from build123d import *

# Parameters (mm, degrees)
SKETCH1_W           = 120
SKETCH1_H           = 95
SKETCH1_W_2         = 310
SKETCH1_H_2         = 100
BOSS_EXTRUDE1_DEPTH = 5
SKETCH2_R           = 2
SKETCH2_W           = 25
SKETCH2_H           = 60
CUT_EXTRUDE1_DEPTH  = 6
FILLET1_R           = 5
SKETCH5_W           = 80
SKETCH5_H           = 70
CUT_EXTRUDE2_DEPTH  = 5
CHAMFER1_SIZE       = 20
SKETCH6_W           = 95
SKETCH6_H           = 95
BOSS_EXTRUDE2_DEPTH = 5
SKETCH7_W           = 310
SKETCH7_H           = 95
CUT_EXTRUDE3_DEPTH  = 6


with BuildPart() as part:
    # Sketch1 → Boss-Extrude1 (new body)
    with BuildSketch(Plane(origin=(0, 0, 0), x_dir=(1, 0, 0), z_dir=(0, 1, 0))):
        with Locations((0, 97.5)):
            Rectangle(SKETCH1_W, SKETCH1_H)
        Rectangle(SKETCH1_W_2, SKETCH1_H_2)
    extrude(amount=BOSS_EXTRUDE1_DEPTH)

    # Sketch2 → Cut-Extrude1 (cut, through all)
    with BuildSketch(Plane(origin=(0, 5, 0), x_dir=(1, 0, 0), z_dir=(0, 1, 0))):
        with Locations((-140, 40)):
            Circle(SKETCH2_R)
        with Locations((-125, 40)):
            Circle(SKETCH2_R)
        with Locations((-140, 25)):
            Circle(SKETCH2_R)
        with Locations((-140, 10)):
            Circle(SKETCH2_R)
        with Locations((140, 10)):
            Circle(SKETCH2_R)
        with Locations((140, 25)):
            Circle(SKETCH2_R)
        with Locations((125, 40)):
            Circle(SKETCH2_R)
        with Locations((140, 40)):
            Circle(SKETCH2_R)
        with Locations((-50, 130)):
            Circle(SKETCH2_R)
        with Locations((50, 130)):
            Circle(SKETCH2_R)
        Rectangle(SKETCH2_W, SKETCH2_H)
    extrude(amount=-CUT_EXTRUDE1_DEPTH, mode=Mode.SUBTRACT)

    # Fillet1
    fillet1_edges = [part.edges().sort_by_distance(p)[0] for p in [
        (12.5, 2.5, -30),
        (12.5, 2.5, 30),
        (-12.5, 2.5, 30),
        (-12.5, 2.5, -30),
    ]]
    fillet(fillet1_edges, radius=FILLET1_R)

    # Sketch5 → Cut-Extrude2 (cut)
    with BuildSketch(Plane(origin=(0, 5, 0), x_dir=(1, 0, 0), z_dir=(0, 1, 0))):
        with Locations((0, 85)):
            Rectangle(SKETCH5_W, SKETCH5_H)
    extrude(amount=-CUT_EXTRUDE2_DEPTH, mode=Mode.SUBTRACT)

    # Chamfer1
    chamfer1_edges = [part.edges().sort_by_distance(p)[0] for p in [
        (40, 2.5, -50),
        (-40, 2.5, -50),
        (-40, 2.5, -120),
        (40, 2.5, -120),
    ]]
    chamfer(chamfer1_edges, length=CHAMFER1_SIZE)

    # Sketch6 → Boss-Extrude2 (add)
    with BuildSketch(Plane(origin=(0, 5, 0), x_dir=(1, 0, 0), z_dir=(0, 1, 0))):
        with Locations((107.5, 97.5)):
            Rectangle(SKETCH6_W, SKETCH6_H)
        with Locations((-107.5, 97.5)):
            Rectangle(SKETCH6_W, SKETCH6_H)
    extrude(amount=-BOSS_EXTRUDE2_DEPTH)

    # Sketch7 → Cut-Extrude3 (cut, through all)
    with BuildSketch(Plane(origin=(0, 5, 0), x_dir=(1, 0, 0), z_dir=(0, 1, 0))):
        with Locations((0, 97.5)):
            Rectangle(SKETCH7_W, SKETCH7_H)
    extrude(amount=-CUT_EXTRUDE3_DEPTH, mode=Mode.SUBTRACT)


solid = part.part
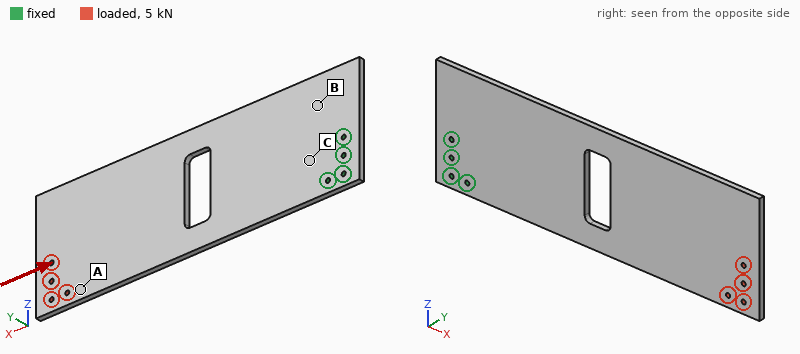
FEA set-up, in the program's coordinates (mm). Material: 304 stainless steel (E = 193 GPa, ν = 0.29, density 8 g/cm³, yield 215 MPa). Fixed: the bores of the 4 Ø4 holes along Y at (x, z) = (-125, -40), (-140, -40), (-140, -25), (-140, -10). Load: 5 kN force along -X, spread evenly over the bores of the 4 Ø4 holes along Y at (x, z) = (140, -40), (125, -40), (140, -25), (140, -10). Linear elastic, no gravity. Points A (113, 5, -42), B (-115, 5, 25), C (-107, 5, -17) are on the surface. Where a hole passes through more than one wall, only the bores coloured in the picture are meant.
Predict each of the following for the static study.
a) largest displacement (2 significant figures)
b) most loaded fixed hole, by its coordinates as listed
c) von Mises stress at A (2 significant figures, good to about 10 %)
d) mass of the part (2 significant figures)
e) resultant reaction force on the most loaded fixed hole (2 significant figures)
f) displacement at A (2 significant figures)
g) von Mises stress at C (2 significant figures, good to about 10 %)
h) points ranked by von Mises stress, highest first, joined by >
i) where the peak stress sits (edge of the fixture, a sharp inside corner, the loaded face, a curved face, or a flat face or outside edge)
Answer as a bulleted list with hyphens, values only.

- 82 µm
- (-125, -40)
- 26 MPa
- 1.2 kg
- 2.1 kN
- 63 µm
- 15 MPa
- A > C > B
- a curved face
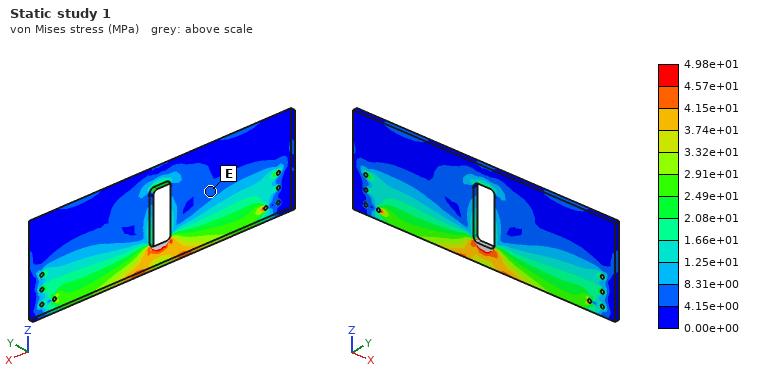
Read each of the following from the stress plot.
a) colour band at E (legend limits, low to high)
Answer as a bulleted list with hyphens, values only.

- 4.15e+00 to 8.31e+00 MPa
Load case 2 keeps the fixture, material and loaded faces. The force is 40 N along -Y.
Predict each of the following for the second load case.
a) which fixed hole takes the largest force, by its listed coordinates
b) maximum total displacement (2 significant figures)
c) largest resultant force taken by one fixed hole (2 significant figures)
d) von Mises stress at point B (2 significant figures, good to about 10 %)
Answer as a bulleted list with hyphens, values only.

- (-125, -40)
- 1.8 mm
- 240 N
- 17 MPa
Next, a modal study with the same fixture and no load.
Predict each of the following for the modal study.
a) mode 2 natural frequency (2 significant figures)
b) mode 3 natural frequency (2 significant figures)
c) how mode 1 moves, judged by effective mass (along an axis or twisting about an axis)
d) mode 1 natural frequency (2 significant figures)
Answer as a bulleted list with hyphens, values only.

- 230 Hz
- 280 Hz
- along Y
- 43 Hz
